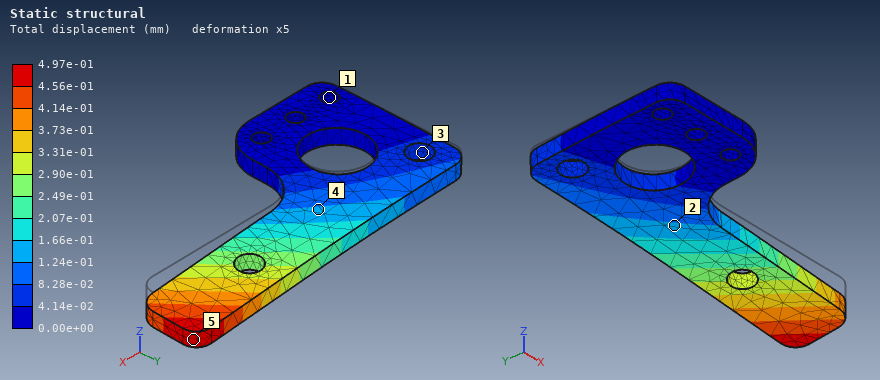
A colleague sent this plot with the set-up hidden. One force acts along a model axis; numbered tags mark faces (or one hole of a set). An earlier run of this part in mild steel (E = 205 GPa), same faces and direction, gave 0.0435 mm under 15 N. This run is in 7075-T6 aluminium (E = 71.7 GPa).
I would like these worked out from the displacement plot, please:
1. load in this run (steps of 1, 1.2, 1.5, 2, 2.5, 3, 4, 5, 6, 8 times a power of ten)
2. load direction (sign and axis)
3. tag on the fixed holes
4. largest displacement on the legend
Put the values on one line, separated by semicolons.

60 N; -Z; 1; 4.97e-01 mm
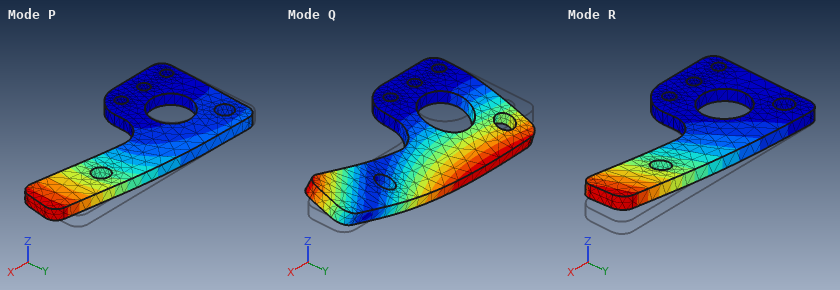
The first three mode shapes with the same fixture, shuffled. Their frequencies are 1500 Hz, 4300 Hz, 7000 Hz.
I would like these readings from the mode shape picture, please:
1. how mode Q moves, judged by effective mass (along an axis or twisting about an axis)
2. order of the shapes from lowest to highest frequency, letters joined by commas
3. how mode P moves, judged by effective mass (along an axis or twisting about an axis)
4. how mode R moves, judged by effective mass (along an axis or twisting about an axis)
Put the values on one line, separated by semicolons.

along Z; R, Q, P; along Y; along Z
